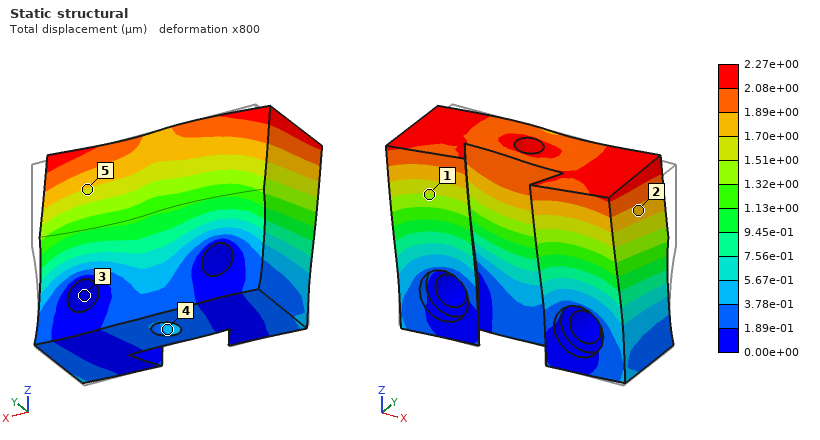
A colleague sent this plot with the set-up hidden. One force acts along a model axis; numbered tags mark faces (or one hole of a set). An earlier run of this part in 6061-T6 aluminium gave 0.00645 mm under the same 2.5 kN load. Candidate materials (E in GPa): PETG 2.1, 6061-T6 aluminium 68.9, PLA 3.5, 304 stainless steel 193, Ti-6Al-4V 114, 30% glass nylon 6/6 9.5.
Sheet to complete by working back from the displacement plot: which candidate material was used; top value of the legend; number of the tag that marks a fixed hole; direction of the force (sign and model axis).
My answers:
304 stainless steel
2.27e+00 µm
3
-X
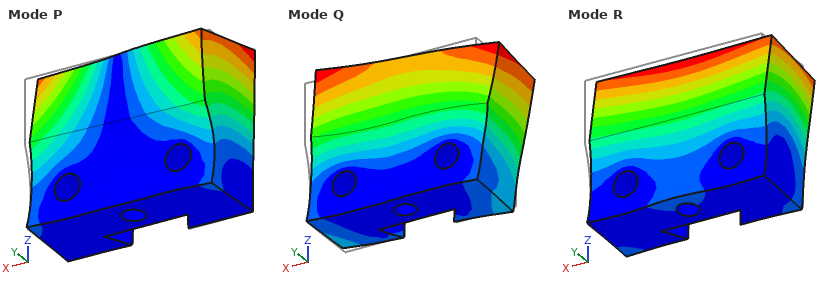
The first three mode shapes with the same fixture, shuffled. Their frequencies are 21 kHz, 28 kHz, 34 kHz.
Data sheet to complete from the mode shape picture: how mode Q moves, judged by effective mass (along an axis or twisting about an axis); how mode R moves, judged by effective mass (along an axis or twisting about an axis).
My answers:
along X
along Y
